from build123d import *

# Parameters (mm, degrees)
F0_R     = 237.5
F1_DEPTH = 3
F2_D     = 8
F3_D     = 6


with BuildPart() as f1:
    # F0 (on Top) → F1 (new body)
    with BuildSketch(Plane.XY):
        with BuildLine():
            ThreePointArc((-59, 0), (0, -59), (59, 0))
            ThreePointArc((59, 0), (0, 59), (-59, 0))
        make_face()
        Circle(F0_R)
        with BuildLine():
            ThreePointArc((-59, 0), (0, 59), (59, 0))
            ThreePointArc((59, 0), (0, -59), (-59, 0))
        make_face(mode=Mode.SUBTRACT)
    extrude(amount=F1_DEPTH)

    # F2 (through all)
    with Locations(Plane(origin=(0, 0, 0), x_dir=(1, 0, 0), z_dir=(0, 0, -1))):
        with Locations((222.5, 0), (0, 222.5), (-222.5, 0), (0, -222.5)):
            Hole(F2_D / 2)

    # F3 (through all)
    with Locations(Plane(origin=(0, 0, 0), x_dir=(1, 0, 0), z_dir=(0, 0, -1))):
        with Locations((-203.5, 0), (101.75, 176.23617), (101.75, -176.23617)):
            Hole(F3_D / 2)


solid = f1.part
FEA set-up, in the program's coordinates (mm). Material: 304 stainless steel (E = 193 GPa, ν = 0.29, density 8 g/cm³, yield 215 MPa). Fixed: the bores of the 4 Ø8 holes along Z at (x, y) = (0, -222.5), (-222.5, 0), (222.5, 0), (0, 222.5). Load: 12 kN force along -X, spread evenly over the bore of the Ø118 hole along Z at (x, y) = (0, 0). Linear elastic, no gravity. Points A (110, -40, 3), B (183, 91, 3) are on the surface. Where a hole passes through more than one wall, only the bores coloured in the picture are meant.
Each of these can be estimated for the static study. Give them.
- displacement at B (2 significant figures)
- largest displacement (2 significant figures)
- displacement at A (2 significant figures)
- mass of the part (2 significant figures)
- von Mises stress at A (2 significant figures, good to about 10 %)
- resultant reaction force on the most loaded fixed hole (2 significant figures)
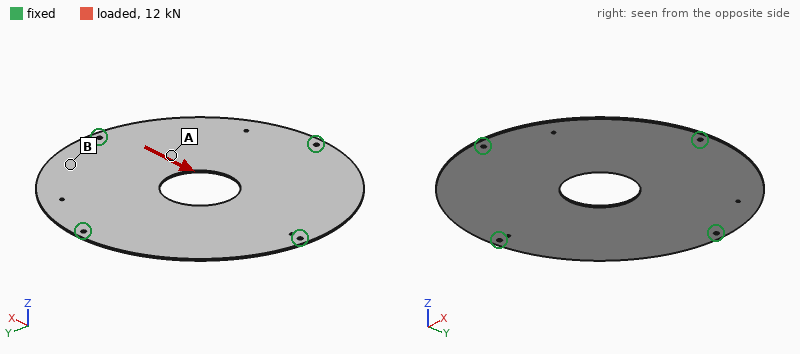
9.3 µm
16 µm
11 µm
4.0 kg
11 MPa
3.6 kN
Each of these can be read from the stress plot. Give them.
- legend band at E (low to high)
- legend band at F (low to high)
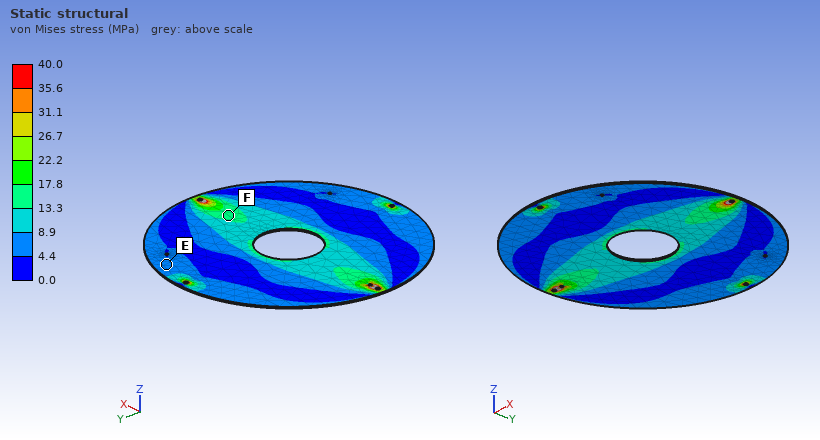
4.4 to 8.9 MPa
13.3 to 17.8 MPa
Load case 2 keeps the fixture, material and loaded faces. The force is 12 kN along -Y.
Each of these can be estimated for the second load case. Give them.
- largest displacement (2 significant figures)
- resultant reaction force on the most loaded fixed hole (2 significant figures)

16 µm
3.6 kN
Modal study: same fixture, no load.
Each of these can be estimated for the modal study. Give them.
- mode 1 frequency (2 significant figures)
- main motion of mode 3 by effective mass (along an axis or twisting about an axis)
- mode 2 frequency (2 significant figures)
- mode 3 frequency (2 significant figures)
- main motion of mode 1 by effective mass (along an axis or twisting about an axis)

100 Hz
twisting about Y
120 Hz
130 Hz
along Z
